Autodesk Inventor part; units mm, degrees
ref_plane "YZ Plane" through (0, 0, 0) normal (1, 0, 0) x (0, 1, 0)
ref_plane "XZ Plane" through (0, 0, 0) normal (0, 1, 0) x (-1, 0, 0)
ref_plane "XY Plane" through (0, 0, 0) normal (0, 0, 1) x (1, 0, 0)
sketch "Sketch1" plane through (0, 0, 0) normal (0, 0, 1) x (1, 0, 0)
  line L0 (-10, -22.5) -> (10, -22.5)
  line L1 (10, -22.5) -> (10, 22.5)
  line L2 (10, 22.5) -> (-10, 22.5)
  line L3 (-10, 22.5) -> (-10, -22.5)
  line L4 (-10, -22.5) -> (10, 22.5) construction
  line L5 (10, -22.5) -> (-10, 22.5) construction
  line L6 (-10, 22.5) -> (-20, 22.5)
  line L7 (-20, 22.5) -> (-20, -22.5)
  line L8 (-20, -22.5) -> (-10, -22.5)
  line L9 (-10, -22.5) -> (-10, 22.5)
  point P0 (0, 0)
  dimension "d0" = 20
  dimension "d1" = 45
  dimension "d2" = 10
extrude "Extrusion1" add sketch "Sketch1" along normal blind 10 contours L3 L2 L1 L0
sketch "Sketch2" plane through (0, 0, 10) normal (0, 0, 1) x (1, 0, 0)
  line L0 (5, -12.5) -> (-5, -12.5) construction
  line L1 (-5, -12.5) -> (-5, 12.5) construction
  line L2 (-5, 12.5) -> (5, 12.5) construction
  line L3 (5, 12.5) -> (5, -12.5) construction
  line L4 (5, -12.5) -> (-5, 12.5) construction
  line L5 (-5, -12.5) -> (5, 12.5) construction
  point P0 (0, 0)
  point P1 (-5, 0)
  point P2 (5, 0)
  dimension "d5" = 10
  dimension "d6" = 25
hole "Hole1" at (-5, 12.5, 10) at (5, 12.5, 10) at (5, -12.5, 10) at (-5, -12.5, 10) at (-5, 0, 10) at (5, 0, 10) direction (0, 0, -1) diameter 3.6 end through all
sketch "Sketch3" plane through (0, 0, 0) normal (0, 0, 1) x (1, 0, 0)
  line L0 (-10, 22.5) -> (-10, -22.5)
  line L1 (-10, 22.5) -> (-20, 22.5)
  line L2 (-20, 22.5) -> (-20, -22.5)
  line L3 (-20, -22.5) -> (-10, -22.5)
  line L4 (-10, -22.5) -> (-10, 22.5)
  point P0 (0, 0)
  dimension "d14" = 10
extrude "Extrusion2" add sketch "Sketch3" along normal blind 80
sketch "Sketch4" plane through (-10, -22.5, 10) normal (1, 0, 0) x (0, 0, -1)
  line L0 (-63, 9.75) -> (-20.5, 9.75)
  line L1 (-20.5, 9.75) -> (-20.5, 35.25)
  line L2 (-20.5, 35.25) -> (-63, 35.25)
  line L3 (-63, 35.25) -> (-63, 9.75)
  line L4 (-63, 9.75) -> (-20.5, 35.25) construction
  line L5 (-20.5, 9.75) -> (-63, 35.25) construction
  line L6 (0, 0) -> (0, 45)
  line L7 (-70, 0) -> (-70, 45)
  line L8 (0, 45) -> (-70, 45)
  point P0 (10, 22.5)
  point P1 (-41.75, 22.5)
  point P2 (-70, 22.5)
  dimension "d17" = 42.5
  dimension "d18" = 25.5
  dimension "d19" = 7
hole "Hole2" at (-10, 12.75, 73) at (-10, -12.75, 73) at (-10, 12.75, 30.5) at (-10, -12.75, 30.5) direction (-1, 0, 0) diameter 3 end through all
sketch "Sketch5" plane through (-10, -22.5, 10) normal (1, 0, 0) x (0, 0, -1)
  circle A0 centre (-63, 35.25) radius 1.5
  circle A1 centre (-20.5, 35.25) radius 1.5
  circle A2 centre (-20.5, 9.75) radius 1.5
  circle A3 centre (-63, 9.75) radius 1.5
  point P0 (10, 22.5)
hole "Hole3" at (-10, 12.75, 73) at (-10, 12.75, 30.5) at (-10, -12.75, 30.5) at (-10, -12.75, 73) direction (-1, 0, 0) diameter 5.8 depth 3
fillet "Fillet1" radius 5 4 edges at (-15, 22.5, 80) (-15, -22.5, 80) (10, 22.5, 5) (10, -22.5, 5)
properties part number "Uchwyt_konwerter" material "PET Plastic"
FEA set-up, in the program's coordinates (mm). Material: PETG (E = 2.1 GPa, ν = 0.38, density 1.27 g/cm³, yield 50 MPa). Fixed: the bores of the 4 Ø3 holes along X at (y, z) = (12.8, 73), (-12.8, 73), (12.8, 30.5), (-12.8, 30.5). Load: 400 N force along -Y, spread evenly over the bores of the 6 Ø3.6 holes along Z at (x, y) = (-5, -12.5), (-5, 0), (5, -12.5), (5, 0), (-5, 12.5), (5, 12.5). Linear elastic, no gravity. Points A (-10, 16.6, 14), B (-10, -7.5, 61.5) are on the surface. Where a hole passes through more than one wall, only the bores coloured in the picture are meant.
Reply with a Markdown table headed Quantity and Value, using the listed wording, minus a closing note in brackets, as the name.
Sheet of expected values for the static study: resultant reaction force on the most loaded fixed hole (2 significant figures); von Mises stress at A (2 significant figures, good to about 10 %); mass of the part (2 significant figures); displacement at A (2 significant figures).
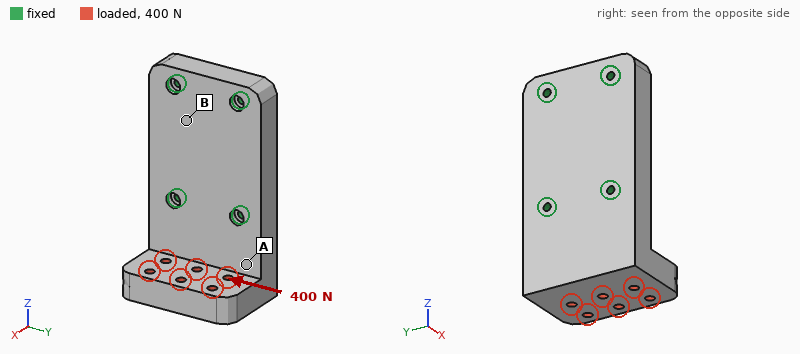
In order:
| Quantity | Value |
|---|---|
| resultant reaction force on the most loaded fixed hole | 440 N |
| von Mises stress at A | 5.6 MPa |
| mass of the part | 55 g |
| displacement at A | 0.13 mm |
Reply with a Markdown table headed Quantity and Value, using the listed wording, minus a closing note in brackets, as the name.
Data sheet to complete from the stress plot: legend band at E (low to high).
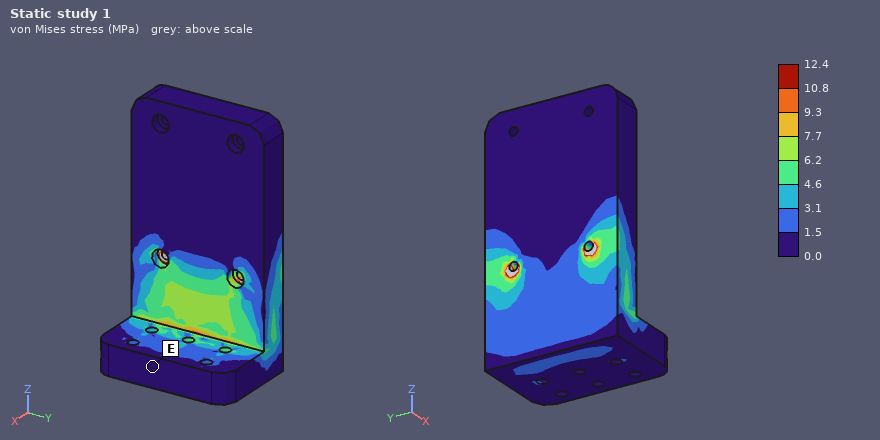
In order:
| Quantity | Value |
|---|---|
| legend band at E | 0.0 to 1.5 MPa |
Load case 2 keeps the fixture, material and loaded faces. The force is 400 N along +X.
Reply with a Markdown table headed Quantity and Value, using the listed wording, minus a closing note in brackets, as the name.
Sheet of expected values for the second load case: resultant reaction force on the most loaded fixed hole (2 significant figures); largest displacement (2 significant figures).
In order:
| Quantity | Value |
|---|---|
| resultant reaction force on the most loaded fixed hole | 290 N |
| largest displacement | 0.89 mm |
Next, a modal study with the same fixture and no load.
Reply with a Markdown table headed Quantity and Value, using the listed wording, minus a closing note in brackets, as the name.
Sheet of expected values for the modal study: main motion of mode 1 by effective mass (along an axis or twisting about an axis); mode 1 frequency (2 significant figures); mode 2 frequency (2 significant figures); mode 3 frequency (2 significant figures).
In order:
| Quantity | Value |
|---|---|
| main motion of mode 1 by effective mass | along X |
| mode 1 frequency | 880 Hz |
| mode 2 frequency | 1600 Hz |
| mode 3 frequency | 2800 Hz |
